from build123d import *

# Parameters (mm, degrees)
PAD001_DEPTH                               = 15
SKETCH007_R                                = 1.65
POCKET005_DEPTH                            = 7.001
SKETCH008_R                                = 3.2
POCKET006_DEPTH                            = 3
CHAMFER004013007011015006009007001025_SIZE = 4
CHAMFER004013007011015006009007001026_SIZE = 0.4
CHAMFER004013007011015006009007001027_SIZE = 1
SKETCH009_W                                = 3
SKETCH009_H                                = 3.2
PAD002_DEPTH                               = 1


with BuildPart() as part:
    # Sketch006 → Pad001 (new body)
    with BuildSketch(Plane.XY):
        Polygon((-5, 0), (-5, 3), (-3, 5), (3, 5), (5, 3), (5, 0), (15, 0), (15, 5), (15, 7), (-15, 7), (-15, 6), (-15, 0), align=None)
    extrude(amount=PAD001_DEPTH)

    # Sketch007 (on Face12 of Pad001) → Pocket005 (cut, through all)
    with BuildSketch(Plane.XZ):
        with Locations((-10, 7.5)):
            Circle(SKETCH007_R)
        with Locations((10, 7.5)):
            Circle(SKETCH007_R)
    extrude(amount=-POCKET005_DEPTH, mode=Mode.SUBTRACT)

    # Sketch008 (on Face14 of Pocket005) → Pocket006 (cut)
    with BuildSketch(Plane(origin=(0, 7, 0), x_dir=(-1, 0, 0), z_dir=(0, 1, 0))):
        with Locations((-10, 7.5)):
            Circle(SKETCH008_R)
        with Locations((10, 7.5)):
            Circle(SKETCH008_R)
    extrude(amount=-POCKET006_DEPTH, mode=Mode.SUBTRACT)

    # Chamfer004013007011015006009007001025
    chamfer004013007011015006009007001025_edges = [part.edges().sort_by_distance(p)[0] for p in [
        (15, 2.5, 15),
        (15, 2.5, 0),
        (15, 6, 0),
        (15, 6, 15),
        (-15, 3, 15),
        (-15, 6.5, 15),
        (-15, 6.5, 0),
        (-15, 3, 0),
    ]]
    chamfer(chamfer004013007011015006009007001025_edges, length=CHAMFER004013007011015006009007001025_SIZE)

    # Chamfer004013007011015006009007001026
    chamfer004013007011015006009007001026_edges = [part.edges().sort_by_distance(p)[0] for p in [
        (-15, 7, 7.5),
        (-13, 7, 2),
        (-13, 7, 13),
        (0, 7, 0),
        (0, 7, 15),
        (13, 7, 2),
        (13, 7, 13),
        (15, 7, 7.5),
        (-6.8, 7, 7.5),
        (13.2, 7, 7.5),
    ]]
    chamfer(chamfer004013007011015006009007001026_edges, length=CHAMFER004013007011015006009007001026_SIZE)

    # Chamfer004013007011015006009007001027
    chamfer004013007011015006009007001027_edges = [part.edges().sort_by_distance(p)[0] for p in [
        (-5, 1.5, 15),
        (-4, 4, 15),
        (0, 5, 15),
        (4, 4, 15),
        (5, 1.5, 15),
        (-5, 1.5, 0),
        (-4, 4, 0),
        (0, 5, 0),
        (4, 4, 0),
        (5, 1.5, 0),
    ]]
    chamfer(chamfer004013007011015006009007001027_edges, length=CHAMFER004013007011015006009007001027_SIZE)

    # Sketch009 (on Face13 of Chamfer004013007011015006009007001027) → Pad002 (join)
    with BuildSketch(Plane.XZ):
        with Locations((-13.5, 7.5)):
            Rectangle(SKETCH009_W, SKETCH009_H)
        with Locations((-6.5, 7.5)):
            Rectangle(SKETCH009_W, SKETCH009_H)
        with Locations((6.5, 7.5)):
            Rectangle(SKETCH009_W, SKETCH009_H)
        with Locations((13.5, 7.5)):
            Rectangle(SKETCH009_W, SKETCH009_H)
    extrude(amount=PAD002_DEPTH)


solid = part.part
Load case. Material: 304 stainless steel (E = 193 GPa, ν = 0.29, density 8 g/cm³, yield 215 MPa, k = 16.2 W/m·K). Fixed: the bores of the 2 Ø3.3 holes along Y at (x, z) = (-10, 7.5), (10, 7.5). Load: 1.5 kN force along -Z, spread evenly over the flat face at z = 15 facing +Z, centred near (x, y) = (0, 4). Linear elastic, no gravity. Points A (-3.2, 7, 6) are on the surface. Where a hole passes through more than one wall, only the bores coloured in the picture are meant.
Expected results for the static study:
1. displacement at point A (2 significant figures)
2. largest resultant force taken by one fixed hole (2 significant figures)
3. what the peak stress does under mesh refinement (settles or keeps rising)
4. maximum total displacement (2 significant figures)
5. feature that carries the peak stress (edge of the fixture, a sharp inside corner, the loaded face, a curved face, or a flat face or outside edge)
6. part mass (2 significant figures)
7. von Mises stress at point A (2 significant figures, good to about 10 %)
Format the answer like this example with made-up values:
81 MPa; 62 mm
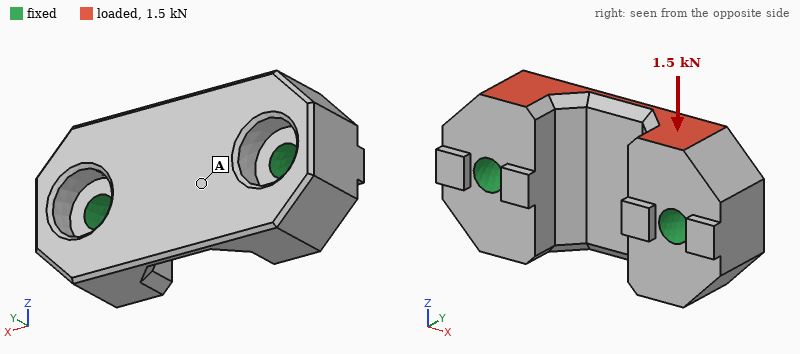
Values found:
1.8 µm; 750 N; keeps rising; 3.1 µm; edge of the fixture; 16 g; 11 MPa
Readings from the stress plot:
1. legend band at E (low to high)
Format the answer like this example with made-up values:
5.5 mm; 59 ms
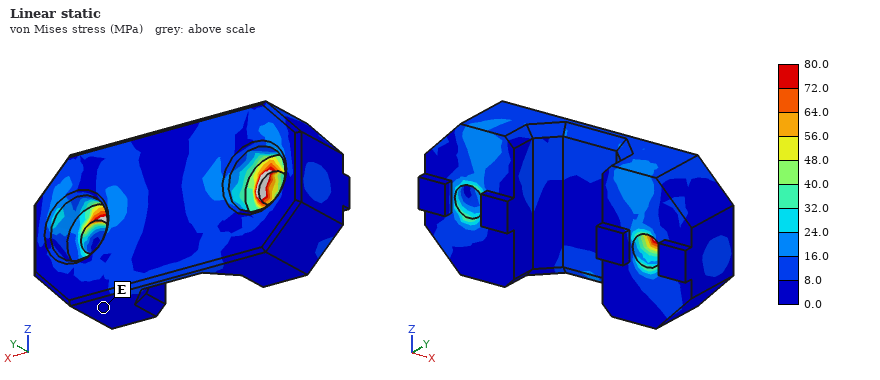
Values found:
0.0 to 8.0 MPa
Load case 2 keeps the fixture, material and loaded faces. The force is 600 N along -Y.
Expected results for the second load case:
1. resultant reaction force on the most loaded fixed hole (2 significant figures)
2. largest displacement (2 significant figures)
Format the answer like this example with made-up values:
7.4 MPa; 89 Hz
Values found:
310 N; 4.0 µm
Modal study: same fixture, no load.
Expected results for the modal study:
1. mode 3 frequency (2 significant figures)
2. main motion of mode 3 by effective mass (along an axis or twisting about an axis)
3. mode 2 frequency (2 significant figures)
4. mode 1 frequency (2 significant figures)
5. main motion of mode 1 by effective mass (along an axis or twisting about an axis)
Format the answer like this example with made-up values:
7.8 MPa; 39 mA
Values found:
50 kHz; along Y; 41 kHz; 32 kHz; along Z
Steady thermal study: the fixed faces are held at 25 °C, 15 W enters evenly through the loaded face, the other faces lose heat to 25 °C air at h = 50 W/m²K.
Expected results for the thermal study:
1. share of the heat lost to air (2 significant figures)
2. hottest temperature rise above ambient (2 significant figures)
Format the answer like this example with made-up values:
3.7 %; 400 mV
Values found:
9.6 %; 68 K
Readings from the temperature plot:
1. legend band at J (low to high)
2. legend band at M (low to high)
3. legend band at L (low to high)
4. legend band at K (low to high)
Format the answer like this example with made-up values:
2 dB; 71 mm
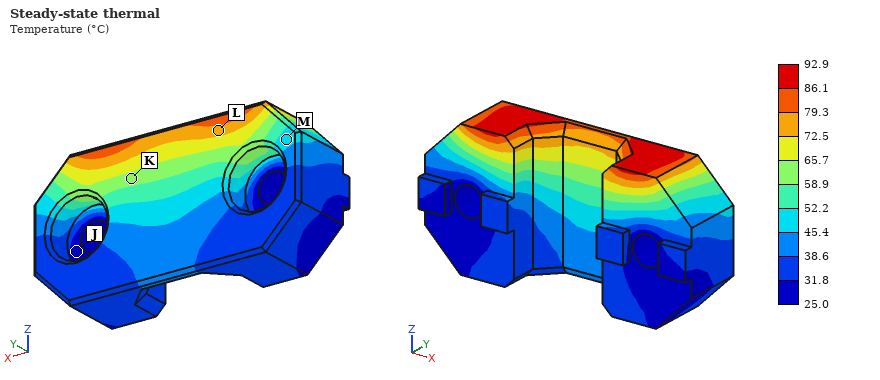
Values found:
25.0 to 31.8 °C; 45.4 to 52.2 °C; 72.5 to 79.3 °C; 58.9 to 65.7 °C
